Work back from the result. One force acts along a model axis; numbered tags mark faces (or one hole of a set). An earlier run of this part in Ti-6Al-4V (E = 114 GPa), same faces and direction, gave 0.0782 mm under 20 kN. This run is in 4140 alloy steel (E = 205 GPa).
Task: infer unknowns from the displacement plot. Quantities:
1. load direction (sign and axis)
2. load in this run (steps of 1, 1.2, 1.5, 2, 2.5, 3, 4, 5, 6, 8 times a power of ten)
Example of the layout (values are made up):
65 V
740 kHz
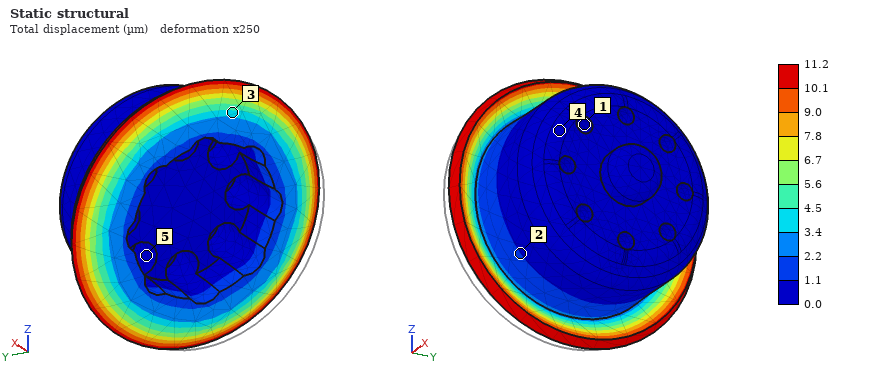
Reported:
+X
5 kN
